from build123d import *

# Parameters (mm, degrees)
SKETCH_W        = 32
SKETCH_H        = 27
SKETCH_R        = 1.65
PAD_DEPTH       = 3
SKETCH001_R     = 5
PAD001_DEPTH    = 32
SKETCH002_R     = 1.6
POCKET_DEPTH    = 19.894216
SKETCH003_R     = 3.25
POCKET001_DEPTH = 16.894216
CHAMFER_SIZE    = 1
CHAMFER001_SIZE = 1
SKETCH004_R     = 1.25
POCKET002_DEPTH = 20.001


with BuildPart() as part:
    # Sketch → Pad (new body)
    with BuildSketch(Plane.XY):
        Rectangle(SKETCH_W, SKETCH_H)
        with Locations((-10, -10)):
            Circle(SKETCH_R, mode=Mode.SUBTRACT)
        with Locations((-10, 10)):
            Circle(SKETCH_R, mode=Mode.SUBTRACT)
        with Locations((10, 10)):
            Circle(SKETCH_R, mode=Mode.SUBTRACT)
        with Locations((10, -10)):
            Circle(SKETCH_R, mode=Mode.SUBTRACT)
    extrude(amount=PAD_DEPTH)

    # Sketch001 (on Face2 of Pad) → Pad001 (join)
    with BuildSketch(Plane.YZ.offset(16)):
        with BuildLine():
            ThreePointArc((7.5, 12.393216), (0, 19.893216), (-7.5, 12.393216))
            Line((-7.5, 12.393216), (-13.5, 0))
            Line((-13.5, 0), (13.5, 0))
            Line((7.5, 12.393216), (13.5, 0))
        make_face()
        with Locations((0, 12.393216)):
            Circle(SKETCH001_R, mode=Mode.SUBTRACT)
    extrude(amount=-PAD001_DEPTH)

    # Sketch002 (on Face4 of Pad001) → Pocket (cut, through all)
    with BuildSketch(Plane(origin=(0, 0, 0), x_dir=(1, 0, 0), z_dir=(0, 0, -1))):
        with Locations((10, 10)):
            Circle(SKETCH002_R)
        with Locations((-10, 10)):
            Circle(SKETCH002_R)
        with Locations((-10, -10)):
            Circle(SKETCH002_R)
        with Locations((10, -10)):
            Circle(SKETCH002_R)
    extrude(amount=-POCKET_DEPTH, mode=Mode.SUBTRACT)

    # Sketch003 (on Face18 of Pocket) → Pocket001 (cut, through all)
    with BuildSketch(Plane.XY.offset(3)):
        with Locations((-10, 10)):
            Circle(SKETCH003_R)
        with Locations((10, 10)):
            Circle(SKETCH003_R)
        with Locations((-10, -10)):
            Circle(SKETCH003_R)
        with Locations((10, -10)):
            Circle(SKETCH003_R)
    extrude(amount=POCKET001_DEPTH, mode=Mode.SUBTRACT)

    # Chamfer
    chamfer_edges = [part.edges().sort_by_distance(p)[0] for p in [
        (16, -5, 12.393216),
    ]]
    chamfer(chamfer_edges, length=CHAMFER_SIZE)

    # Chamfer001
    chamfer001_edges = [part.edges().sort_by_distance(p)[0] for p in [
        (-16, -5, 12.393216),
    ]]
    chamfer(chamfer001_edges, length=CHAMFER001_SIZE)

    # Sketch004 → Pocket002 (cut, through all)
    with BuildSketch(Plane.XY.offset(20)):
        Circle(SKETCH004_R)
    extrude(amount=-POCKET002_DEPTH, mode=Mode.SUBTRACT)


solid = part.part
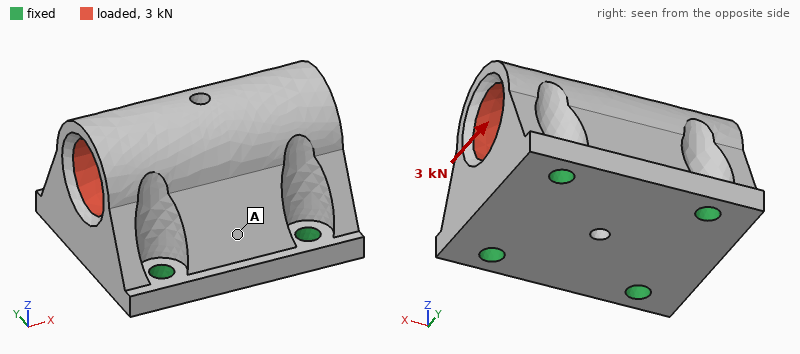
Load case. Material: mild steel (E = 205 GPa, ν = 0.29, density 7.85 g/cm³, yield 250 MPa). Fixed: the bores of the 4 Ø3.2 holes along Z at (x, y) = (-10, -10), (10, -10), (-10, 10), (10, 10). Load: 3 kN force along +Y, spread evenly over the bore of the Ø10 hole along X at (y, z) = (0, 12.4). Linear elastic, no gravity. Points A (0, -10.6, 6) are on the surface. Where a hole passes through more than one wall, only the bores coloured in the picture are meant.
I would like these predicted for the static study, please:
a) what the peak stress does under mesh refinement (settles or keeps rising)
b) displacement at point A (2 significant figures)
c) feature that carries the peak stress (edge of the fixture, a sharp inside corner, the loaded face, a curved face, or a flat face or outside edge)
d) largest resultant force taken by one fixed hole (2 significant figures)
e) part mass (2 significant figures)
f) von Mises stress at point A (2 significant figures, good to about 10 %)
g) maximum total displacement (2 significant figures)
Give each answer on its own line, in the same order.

keeps rising
2.5 µm
edge of the fixture
1.1 kN
63 g
11 MPa
7.4 µm
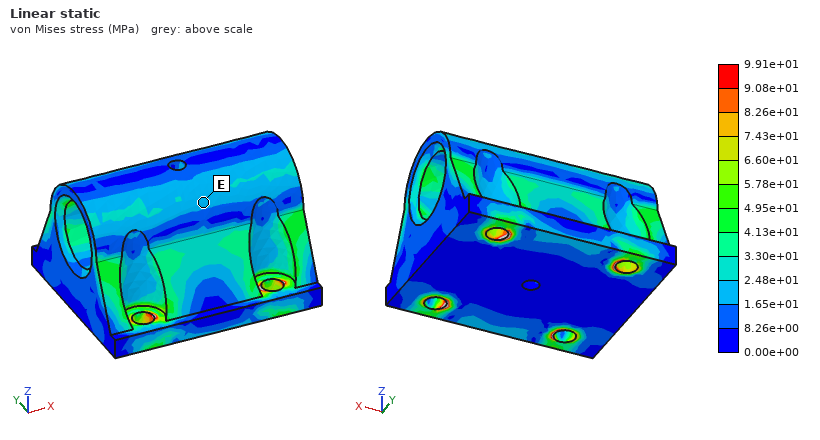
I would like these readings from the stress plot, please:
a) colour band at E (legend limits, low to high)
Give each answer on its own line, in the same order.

1.65e+01 to 2.48e+01 MPa
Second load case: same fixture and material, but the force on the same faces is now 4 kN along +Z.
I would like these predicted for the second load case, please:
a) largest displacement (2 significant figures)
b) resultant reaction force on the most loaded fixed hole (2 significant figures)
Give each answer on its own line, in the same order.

3.1 µm
1.1 kN
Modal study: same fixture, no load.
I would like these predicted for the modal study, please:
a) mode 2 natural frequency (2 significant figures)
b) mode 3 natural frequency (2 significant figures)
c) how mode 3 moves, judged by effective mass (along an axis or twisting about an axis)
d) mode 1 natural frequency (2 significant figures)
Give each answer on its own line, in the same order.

23 kHz
29 kHz
along Z
22 kHz
